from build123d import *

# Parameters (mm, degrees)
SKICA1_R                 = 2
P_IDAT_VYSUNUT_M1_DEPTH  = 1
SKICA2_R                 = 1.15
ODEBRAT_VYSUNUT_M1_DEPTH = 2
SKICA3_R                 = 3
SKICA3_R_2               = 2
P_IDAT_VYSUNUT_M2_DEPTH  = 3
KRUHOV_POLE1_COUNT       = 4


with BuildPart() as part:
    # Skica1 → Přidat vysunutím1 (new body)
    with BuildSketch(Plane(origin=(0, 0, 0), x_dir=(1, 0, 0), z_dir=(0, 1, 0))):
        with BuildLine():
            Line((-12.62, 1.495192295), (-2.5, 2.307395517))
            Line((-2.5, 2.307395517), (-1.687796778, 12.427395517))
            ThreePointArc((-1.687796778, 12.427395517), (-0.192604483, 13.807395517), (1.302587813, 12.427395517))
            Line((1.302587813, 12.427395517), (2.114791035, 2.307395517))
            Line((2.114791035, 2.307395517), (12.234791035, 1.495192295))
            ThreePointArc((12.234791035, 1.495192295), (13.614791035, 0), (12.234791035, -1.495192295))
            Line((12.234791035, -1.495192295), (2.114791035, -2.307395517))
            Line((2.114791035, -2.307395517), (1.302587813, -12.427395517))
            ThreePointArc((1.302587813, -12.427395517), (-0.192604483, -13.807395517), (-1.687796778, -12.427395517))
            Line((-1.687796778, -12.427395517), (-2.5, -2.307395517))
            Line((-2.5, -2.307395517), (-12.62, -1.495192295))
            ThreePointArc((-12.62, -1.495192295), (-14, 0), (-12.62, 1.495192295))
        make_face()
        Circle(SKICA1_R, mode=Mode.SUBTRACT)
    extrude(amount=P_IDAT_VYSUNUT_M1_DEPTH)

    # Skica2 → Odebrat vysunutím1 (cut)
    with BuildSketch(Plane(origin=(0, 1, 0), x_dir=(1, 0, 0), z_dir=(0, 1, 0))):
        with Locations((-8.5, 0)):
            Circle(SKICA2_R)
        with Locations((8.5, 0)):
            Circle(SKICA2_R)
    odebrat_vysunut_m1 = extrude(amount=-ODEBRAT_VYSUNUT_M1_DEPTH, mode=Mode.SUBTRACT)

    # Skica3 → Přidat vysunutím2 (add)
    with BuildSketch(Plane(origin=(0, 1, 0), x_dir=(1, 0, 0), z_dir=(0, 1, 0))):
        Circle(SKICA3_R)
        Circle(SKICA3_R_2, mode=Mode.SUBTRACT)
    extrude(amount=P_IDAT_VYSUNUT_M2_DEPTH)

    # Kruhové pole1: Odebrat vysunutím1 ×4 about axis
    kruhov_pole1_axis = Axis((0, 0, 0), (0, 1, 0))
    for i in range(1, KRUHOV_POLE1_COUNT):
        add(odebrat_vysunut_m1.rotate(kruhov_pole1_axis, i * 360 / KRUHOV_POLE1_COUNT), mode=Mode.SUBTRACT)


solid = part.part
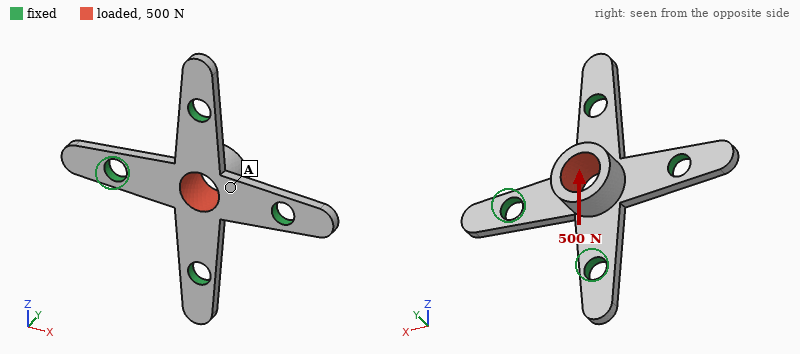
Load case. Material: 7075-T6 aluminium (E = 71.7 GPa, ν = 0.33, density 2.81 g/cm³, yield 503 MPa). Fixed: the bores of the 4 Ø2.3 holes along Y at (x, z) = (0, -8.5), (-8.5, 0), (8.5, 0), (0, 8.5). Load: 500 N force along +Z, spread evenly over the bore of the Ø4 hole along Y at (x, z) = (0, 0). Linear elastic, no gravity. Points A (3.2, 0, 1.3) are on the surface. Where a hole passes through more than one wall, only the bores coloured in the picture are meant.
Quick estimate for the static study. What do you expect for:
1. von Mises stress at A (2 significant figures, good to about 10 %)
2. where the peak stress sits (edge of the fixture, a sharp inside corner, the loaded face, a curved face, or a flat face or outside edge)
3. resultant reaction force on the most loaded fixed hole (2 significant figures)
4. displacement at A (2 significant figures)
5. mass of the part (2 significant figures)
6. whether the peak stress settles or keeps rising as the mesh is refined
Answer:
29 MPa
edge of the fixture
230 N
7.4 µm
0.58 g
keeps rising
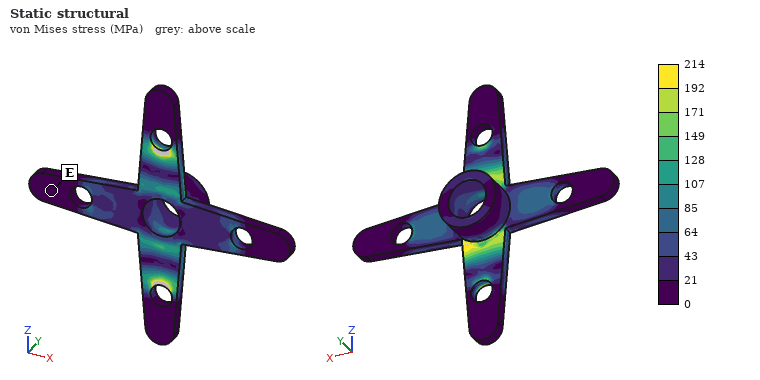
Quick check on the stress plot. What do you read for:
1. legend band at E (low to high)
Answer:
0 to 21 MPa
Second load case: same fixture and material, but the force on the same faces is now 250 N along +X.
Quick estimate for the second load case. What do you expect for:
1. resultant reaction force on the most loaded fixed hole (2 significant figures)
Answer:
110 N
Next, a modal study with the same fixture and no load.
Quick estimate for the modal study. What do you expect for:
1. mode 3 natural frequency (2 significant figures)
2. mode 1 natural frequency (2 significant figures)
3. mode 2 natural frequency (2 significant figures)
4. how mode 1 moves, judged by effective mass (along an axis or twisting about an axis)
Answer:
41 kHz
26 kHz
41 kHz
along Y
